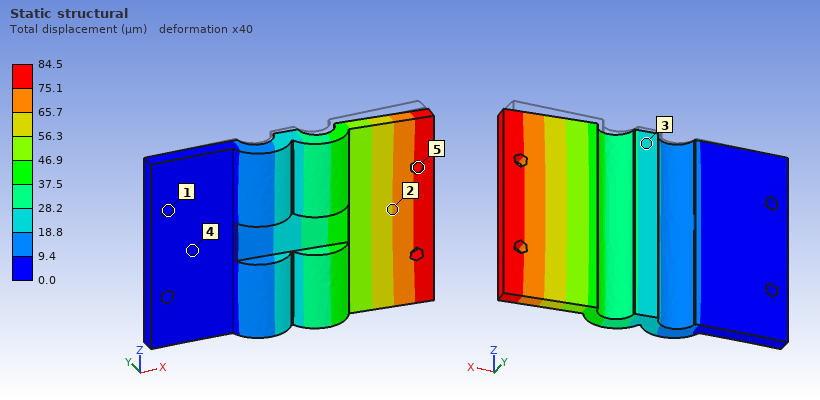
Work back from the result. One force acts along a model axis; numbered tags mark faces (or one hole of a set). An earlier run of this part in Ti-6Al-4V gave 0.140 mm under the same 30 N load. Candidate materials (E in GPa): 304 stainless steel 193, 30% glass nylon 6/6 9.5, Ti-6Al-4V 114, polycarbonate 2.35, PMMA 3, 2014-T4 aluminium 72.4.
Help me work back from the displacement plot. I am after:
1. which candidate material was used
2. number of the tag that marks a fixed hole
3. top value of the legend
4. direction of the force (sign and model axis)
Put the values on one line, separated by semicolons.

304 stainless steel; 1; 84.5 µm; -Y
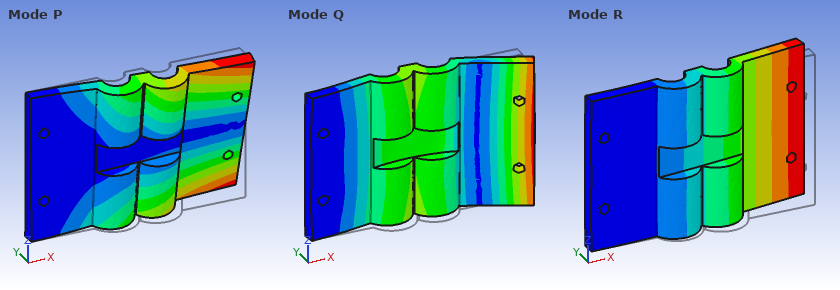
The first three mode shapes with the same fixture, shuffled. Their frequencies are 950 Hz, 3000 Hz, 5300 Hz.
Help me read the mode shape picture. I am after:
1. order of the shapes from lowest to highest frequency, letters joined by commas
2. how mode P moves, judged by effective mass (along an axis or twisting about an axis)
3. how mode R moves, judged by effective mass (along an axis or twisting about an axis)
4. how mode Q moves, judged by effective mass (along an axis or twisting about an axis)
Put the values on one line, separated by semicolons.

R, P, Q; twisting about X; along Y; along Y
